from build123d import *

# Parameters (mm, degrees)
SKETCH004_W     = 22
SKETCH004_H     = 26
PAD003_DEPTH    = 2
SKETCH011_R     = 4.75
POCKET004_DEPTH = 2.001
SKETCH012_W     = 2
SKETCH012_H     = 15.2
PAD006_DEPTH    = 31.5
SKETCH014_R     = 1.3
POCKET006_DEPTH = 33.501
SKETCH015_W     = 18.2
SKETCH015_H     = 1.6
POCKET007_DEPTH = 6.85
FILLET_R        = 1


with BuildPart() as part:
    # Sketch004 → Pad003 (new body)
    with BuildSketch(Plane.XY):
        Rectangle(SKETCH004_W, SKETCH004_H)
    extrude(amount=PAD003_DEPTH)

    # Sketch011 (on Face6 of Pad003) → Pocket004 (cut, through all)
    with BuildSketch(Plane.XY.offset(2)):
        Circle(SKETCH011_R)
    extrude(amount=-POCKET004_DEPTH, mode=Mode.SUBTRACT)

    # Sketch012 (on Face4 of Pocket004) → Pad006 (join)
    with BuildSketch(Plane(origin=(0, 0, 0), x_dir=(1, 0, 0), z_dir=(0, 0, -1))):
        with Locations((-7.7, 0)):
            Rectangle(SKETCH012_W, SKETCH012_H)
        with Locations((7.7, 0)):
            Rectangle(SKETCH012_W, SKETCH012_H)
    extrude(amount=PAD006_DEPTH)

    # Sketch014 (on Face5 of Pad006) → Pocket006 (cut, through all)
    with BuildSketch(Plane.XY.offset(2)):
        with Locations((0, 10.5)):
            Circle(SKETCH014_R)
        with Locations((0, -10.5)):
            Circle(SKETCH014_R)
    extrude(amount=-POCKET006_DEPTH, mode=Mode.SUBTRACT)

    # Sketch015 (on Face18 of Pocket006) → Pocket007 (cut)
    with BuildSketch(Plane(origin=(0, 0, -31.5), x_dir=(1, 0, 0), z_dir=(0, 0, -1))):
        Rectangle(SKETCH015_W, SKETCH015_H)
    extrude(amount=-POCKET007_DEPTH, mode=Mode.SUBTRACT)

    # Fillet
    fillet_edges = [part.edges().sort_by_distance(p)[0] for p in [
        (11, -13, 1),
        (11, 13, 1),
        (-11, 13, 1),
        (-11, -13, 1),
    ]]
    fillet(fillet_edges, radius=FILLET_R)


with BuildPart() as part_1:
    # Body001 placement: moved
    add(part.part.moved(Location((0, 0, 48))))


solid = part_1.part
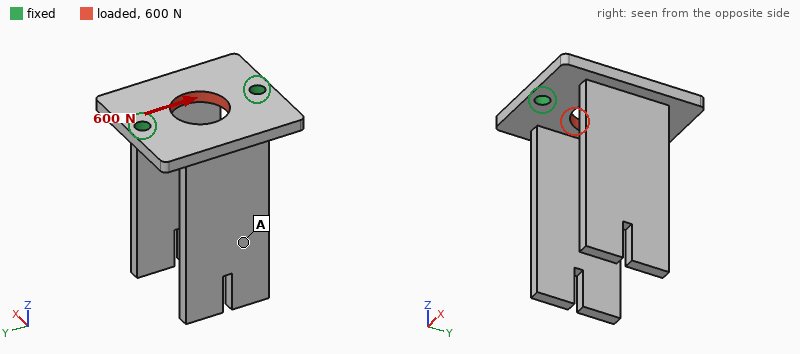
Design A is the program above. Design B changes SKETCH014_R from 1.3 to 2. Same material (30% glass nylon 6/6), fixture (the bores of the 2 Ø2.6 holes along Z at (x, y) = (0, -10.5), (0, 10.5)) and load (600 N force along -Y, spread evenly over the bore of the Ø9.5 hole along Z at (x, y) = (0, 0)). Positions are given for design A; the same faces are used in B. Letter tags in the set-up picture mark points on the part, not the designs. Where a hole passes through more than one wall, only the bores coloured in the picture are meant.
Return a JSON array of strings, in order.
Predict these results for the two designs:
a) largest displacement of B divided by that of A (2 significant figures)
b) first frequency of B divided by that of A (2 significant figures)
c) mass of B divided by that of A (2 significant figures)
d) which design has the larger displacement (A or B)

["0.84", "1.0", "0.99", "A"]
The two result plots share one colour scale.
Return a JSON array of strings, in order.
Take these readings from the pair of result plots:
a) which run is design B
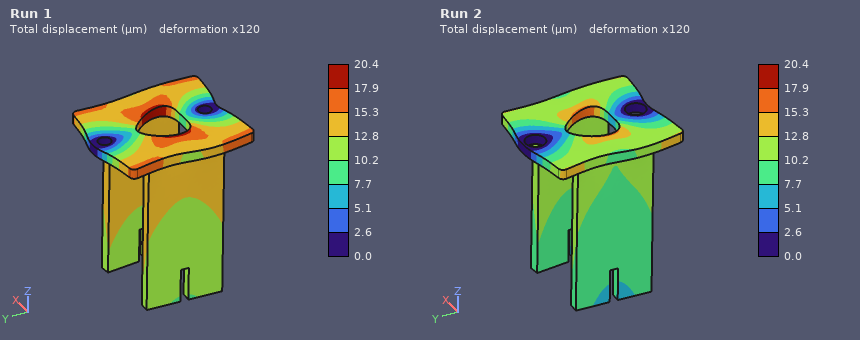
["Run 2"]
